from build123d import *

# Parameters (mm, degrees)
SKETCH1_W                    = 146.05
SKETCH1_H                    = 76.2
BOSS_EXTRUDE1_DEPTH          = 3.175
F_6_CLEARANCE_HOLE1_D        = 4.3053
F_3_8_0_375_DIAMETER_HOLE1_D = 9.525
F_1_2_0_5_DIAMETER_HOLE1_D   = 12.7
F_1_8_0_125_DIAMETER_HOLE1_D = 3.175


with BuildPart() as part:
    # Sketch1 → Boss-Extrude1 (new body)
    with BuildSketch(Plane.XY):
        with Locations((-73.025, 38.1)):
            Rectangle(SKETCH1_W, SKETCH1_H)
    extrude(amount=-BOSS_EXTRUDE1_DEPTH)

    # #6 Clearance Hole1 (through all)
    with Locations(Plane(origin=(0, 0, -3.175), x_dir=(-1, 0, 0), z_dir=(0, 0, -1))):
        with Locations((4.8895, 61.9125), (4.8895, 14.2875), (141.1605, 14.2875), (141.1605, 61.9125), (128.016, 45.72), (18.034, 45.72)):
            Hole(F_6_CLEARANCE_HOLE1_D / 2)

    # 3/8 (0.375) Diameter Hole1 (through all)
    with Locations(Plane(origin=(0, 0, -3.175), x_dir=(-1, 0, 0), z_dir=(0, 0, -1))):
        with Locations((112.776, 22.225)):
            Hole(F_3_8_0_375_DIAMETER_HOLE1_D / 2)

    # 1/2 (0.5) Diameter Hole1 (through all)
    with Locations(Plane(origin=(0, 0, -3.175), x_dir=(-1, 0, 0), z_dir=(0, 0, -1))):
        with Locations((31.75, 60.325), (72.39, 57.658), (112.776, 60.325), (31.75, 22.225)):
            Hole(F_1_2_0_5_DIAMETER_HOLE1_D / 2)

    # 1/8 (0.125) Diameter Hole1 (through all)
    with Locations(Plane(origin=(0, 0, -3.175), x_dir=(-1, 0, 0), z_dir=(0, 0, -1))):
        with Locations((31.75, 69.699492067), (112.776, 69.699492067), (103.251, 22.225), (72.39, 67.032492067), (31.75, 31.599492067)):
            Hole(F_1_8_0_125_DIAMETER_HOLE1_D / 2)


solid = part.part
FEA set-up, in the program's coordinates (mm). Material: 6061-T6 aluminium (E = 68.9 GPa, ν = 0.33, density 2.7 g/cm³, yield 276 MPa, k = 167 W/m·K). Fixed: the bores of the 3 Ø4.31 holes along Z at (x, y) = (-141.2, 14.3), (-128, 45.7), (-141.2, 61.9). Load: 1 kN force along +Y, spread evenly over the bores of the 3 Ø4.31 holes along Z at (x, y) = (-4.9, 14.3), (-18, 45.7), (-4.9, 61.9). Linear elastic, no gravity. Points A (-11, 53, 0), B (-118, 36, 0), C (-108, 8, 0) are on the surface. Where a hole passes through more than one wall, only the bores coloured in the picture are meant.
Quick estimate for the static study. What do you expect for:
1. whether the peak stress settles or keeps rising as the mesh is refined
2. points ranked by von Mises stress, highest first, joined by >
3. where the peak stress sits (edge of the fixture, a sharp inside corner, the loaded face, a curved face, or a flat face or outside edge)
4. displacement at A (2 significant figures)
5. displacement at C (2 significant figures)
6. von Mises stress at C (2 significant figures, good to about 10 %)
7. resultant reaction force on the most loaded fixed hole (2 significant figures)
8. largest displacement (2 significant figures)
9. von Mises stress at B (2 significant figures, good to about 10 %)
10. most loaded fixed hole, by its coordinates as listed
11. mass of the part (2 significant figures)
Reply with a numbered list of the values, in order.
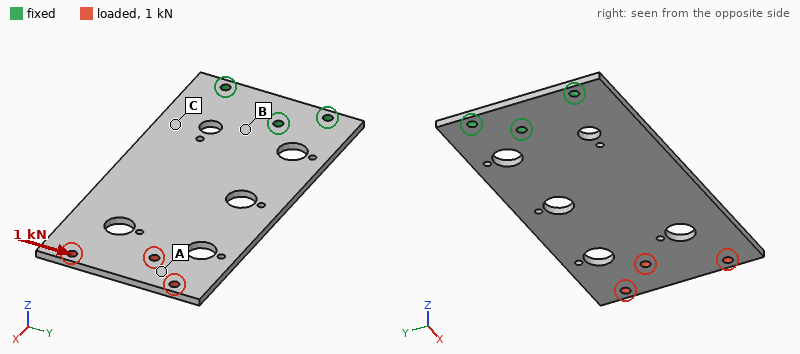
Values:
1. keeps rising
2. C > B > A
3. edge of the fixture
4. 0.16 mm
5. 0.033 mm
6. 29 MPa
7. 2.4 kN
8. 0.19 mm
9. 16 MPa
10. (-141.2, 14.3)
11. 89 g
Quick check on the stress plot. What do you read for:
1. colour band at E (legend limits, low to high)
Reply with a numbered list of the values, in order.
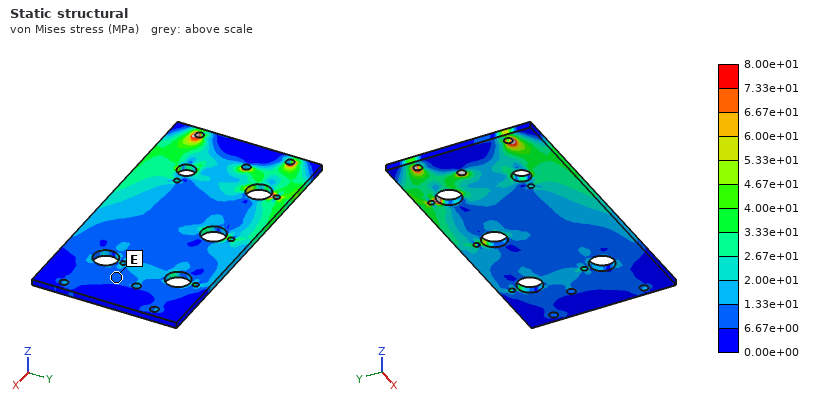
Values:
1. 6.67e+00 to 1.33e+01 MPa
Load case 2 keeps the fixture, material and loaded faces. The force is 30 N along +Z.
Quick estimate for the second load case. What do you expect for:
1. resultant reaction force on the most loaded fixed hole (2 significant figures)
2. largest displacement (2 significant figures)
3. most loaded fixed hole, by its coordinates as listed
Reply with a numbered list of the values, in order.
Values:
1. 120 N
2. 1.6 mm
3. (-128, 45.7)
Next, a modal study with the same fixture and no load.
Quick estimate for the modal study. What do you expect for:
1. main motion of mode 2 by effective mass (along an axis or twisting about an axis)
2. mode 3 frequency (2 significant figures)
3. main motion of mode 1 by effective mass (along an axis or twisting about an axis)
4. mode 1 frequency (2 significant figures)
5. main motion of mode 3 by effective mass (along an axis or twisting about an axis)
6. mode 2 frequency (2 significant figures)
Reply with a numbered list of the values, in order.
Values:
1. twisting about X
2. 890 Hz
3. along Z
4. 150 Hz
5. along Z
6. 520 Hz
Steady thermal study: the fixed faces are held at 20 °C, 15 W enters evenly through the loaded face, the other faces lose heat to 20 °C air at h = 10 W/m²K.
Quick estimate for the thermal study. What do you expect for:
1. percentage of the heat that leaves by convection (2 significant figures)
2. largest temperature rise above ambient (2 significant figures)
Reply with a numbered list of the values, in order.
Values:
1. 31 %
2. 46 K
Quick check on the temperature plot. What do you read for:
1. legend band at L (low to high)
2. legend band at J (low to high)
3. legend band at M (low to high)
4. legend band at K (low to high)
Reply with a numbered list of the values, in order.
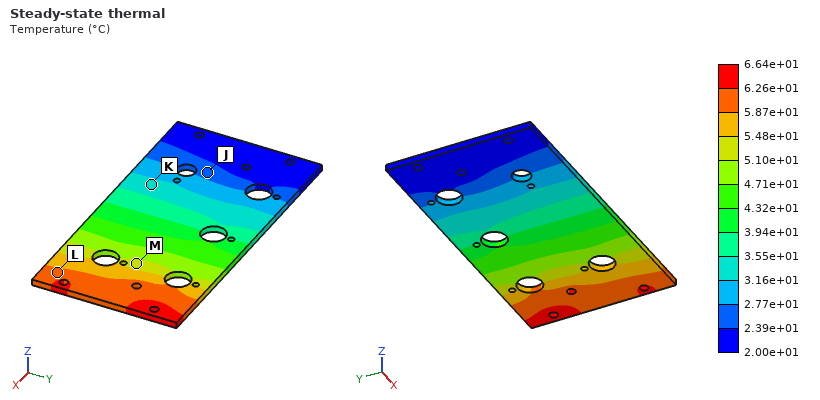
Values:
1. 5.87e+01 to 6.26e+01 °C
2. 2.39e+01 to 2.77e+01 °C
3. 5.10e+01 to 5.48e+01 °C
4. 3.16e+01 to 3.55e+01 °C
